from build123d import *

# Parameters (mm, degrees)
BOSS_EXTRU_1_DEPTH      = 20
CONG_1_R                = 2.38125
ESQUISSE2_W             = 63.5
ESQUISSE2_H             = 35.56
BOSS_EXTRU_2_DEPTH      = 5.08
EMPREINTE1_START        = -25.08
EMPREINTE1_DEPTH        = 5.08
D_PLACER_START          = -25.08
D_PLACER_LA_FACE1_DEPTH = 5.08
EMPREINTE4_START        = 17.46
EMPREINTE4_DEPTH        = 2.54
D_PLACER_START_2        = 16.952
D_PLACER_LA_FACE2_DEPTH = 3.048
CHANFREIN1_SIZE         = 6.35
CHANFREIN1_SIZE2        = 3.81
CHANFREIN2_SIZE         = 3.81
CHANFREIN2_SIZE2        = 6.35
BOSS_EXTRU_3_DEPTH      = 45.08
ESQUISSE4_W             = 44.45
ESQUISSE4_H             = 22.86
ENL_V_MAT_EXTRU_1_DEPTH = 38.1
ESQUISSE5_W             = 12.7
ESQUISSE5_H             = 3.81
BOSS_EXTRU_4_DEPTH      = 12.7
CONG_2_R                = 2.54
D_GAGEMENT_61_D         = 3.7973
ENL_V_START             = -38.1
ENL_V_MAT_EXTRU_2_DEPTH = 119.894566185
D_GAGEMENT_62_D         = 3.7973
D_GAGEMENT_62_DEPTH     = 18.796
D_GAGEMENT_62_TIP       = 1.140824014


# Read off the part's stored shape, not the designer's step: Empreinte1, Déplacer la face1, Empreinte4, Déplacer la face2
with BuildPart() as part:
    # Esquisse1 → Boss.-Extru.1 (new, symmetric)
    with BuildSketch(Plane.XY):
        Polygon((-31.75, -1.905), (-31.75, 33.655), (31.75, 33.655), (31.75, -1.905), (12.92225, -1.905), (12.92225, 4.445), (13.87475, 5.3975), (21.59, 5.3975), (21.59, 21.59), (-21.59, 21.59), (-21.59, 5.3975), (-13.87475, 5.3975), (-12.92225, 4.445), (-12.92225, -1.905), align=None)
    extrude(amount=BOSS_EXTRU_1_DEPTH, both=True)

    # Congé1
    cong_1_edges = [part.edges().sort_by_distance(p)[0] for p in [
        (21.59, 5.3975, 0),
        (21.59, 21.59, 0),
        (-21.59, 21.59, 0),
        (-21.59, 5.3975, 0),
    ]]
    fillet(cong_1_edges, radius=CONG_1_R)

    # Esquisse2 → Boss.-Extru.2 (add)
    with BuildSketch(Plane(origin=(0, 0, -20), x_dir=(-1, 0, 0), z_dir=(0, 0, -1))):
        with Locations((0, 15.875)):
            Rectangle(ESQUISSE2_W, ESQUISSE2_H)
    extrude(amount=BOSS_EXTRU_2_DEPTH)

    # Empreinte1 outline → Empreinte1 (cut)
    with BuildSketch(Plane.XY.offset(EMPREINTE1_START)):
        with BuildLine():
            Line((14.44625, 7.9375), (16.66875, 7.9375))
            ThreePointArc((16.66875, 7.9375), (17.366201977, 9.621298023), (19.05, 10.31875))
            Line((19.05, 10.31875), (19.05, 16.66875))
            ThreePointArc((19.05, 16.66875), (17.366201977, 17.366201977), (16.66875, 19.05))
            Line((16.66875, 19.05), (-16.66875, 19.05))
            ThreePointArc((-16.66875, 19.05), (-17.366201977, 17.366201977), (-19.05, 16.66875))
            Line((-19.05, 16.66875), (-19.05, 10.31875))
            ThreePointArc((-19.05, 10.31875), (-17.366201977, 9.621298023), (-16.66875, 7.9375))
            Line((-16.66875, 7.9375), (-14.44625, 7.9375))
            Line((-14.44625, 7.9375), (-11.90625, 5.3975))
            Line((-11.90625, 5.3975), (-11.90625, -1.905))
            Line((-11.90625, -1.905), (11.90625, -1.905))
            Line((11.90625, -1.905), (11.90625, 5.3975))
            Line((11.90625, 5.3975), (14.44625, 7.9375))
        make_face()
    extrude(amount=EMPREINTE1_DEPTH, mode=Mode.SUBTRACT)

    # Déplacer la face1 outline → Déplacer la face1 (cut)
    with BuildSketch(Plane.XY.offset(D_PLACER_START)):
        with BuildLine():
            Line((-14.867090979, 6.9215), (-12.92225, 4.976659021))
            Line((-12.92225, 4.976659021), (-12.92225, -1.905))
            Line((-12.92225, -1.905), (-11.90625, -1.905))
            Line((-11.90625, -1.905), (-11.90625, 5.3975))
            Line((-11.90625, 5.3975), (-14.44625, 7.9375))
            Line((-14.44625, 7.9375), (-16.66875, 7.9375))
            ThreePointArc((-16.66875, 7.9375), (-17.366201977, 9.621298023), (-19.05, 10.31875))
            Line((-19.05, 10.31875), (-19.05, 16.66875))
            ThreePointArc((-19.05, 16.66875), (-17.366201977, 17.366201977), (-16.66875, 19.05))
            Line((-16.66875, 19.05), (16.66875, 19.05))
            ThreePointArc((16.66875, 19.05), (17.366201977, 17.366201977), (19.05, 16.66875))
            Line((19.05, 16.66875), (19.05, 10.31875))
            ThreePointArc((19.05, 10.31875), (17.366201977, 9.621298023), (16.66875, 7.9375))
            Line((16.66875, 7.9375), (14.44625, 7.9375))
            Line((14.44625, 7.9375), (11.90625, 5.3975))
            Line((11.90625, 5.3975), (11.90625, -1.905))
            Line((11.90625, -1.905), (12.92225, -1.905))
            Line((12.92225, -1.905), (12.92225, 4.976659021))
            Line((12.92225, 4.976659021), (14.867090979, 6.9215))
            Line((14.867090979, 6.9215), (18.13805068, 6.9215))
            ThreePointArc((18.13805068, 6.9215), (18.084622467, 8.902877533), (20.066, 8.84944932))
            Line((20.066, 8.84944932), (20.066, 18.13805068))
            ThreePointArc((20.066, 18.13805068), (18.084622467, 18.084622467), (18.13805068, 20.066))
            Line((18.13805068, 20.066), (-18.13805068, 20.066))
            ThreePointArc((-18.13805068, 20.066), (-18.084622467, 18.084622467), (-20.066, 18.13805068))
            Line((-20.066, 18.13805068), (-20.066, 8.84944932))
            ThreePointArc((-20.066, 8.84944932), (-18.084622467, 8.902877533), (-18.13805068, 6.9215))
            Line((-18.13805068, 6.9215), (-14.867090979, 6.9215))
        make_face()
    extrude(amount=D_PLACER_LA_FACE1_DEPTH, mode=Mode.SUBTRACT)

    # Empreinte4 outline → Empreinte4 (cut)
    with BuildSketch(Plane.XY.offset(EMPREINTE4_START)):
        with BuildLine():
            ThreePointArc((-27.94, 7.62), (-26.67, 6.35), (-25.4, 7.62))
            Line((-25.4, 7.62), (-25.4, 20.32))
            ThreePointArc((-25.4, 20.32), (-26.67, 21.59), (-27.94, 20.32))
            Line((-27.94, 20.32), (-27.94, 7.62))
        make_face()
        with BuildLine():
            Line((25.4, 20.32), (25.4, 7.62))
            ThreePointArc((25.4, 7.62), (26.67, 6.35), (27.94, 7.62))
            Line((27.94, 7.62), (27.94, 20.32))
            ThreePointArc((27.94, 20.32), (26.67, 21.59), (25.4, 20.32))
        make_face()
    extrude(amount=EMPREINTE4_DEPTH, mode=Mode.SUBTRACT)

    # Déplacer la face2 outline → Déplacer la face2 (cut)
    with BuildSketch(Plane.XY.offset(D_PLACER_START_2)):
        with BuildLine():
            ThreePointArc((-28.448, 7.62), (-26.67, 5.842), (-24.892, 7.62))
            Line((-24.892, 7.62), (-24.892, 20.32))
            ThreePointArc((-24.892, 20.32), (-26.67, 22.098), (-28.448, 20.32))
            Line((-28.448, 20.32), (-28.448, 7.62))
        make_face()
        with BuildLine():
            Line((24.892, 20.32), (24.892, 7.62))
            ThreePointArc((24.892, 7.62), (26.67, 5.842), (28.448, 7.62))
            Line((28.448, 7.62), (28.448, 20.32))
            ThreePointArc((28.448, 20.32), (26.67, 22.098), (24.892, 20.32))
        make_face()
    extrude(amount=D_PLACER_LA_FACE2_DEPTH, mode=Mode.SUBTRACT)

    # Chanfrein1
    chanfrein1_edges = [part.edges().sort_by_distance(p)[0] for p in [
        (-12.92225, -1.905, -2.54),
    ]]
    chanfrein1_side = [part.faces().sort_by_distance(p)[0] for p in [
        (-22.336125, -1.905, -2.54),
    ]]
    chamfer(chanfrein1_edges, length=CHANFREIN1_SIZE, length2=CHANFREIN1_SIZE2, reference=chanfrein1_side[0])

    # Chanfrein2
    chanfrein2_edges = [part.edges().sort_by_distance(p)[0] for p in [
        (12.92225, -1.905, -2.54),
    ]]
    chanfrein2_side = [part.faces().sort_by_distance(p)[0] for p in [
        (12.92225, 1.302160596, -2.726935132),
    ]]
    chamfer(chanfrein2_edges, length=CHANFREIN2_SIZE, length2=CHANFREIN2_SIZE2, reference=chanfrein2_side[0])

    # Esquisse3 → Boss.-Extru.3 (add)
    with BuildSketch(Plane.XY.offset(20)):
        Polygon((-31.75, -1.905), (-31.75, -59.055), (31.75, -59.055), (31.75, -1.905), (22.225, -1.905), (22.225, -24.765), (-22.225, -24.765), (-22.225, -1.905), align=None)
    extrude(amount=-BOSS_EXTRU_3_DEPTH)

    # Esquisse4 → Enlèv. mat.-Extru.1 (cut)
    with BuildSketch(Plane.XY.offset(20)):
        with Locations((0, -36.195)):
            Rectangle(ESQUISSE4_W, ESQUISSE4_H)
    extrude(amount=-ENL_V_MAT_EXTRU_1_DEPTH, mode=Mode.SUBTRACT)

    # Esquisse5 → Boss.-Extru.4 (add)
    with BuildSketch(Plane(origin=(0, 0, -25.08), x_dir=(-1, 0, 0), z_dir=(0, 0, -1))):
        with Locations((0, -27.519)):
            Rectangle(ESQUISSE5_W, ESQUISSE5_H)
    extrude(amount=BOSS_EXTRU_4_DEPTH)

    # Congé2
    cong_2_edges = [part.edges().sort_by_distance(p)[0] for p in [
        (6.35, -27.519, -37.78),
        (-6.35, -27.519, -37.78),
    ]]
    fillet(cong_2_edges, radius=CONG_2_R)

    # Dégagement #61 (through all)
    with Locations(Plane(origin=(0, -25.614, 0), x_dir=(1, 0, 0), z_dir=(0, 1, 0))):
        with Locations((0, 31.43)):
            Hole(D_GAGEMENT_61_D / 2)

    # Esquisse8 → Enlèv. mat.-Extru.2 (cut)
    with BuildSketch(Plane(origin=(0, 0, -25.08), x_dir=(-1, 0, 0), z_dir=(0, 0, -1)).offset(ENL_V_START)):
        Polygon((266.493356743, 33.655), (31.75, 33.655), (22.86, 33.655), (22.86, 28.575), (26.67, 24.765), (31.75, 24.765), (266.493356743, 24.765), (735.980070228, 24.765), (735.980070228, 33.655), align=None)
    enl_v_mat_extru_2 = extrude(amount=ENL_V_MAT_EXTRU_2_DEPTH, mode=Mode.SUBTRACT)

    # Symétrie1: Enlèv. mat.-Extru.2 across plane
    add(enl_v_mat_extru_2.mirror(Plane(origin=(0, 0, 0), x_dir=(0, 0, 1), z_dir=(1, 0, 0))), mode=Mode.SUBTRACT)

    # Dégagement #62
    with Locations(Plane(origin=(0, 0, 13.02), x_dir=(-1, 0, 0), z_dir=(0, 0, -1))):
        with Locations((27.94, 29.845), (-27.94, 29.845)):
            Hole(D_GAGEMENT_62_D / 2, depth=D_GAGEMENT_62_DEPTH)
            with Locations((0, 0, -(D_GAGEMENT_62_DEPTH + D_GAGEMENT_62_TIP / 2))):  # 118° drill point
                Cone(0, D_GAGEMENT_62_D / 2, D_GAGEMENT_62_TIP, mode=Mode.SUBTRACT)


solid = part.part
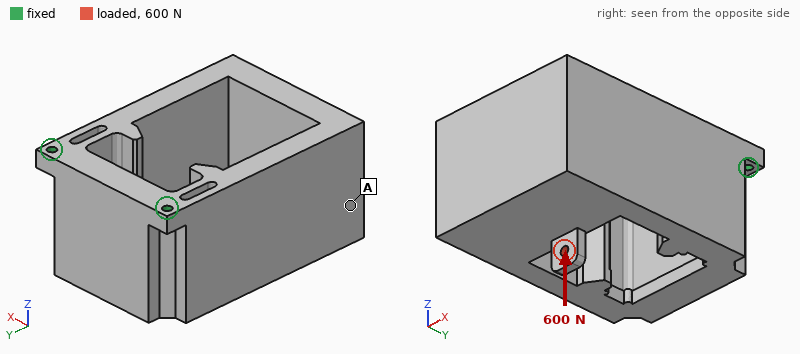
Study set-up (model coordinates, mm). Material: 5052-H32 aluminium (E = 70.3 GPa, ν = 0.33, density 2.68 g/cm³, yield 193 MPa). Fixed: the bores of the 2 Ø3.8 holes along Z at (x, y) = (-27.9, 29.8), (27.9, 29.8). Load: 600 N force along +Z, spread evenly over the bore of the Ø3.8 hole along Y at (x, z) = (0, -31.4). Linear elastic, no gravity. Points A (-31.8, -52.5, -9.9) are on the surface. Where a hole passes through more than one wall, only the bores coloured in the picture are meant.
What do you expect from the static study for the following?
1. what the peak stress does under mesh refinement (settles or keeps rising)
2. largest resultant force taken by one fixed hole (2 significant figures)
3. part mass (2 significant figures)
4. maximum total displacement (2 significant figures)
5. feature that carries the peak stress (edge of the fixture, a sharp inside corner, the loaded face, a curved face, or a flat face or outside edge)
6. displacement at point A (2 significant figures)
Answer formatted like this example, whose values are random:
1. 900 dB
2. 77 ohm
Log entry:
1. keeps rising
2. 360 N
3. 360 g
4. 0.36 mm
5. edge of the fixture
6. 0.32 mm
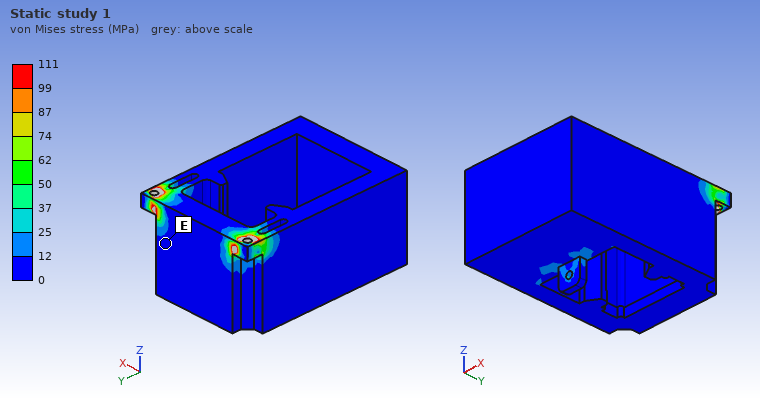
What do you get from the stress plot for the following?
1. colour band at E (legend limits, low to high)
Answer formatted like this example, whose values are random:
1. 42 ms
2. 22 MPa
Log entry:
1. 0 to 12 MPa
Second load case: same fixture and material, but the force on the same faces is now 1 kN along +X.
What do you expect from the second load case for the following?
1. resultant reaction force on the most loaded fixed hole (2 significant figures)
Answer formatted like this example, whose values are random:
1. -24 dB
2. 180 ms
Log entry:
1. 1.4 kN
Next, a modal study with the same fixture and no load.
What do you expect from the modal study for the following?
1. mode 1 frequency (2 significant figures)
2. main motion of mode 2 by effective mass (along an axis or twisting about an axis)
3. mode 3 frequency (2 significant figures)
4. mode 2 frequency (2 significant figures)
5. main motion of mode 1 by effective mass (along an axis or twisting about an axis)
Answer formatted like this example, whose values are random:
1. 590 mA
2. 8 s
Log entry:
1. 430 Hz
2. along X
3. 2800 Hz
4. 1100 Hz
5. along Z
